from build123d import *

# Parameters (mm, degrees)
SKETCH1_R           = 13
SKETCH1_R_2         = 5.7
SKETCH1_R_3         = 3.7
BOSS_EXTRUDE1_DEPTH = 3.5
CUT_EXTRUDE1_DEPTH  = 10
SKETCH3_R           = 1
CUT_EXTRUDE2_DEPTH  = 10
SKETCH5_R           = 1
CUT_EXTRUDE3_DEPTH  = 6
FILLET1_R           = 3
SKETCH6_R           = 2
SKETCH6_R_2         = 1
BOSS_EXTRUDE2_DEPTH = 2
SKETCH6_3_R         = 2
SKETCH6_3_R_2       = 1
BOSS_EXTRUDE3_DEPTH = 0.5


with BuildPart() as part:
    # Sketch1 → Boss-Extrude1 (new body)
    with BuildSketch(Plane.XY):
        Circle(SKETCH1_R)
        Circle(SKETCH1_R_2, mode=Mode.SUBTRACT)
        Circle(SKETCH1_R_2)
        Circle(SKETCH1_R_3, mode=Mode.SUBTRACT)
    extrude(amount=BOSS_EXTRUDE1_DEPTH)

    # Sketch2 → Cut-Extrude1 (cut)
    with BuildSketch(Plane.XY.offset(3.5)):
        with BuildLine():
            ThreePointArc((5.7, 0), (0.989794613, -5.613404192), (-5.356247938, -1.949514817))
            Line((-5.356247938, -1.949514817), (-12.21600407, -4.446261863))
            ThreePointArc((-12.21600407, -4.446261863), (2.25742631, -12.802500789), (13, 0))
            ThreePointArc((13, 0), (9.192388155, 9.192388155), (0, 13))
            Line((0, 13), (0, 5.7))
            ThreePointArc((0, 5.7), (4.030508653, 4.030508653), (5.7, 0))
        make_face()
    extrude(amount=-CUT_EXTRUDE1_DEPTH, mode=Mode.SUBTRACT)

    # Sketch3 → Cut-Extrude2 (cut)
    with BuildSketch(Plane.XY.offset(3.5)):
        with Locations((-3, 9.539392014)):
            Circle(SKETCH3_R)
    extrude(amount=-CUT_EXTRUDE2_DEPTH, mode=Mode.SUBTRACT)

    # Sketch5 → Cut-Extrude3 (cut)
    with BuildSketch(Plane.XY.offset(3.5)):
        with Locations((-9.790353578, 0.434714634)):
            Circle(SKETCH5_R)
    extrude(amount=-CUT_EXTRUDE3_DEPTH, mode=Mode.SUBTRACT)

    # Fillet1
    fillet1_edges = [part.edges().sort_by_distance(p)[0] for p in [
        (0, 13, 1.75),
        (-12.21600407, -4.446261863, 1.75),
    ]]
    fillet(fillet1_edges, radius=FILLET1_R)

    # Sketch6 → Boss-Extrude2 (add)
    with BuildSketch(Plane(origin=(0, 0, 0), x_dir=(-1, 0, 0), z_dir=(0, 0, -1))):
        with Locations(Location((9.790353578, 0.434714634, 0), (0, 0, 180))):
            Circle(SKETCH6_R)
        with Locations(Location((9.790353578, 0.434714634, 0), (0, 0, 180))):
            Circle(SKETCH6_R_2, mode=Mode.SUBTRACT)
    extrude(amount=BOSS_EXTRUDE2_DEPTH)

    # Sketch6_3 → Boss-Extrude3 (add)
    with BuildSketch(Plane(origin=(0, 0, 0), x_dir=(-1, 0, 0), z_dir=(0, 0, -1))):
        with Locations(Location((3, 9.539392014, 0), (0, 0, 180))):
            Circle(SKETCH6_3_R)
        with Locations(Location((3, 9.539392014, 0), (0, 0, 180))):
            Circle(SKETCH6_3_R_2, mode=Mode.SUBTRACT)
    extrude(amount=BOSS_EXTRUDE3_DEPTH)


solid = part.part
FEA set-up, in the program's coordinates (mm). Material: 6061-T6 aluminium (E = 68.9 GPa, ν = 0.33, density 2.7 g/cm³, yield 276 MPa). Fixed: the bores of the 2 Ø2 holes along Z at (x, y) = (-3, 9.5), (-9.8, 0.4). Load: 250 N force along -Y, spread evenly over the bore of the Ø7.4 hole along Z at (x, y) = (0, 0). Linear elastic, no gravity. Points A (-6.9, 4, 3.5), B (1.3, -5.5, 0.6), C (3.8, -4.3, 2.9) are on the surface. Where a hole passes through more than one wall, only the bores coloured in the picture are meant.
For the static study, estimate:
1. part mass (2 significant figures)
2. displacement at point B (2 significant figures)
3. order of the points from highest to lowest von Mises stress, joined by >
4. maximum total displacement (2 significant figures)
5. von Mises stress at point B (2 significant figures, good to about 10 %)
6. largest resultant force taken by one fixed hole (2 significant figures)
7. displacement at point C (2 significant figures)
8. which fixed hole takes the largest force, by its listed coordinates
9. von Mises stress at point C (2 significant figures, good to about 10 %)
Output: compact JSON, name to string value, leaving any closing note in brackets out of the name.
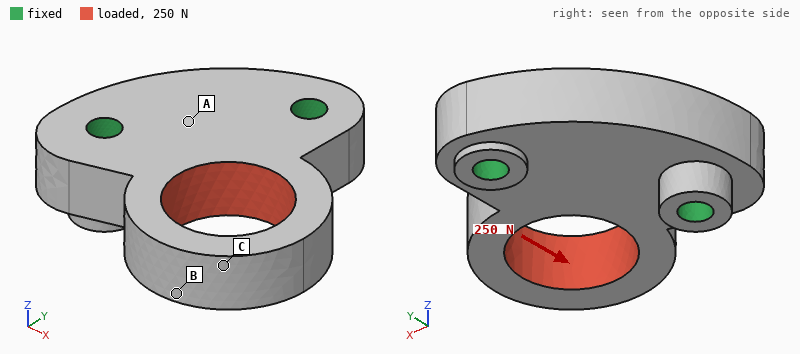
{"part mass": "1.7 g", "displacement at point B": "17 µm", "order of the points from highest to lowest von Mises stress, joined by >": "B > C > A", "maximum total displacement": "18 µm", "von Mises stress at point B": "33 MPa", "largest resultant force taken by one fixed hole": "230 N", "displacement at point C": "17 µm", "which fixed hole takes the largest force, by its listed coordinates": "(-3, 9.5)", "von Mises stress at point C": "21 MPa"}
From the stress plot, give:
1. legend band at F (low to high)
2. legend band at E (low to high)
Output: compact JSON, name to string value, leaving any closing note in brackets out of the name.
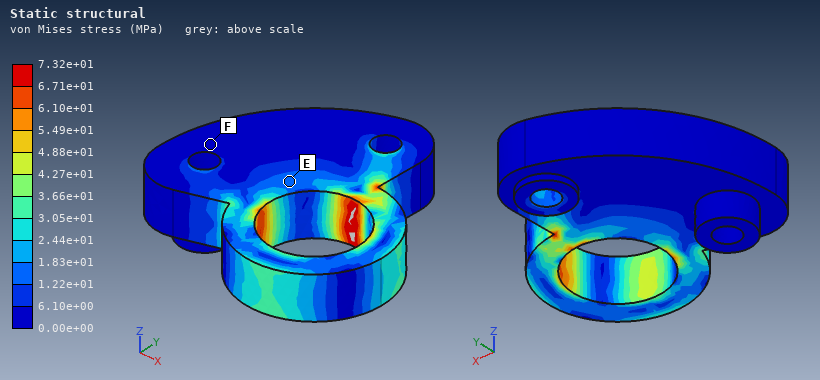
{"legend band at F": "0.00e+00 to 6.10e+00 MPa", "legend band at E": "1.22e+01 to 1.83e+01 MPa"}
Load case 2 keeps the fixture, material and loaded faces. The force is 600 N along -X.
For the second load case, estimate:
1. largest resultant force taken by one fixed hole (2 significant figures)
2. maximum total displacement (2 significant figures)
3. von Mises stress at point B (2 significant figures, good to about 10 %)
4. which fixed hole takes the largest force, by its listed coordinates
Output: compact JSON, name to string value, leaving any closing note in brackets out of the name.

{"largest resultant force taken by one fixed hole": "530 N", "maximum total displacement": "31 µm", "von Mises stress at point B": "42 MPa", "which fixed hole takes the largest force, by its listed coordinates": "(-9.8, 0.4)"}
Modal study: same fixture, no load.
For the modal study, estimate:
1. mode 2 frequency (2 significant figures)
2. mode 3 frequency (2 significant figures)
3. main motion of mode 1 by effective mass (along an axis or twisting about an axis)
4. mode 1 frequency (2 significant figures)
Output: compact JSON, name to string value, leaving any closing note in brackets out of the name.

{"mode 2 frequency": "25 kHz", "mode 3 frequency": "37 kHz", "main motion of mode 1 by effective mass": "along Z", "mode 1 frequency": "17 kHz"}
